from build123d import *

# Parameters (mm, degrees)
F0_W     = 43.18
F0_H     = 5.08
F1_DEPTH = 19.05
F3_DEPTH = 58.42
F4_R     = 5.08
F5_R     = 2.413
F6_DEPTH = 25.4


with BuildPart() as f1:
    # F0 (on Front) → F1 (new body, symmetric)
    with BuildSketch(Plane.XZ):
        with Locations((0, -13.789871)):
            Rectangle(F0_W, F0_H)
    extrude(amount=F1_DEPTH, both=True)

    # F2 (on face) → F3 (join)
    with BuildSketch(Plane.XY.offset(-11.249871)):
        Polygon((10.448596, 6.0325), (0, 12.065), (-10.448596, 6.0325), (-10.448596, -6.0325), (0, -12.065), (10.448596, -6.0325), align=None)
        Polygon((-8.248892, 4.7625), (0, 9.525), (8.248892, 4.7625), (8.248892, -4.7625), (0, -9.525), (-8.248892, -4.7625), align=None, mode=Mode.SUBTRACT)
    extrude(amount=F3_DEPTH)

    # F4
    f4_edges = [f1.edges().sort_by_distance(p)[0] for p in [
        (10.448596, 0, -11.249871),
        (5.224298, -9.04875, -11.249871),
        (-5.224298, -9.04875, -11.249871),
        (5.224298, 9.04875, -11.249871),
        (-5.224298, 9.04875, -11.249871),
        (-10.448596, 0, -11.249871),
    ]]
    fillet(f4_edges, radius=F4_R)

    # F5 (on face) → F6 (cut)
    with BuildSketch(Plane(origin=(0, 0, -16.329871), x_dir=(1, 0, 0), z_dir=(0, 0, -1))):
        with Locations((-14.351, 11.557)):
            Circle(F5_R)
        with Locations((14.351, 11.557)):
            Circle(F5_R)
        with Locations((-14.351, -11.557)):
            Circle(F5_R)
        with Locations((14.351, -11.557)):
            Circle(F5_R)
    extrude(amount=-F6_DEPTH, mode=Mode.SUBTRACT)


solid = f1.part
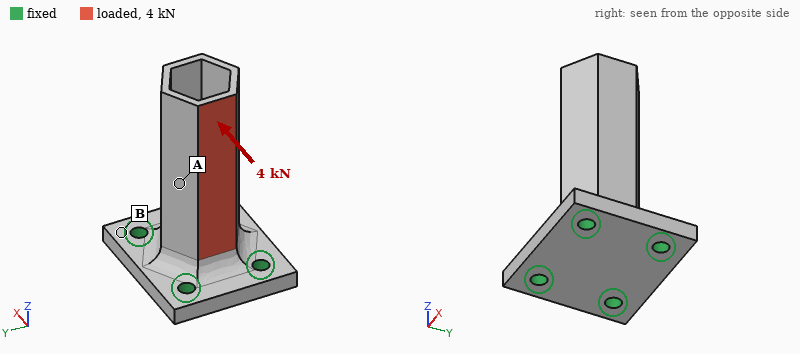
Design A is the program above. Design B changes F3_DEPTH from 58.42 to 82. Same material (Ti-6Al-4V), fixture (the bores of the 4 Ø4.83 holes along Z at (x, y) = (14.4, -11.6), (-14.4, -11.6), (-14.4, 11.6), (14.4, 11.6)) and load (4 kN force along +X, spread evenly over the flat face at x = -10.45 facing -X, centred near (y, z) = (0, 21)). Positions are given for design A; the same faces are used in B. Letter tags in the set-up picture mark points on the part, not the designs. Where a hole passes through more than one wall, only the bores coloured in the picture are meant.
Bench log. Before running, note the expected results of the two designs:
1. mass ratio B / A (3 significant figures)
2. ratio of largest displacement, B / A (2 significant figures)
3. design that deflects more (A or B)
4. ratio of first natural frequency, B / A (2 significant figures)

1.20
2.1
B
0.56
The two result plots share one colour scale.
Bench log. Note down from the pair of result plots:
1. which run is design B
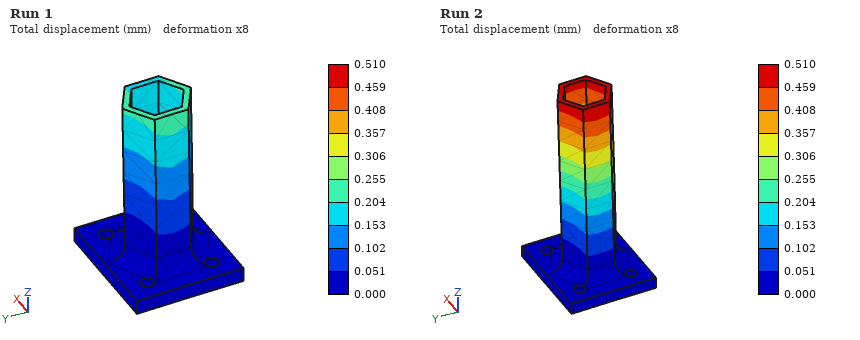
Run 2
